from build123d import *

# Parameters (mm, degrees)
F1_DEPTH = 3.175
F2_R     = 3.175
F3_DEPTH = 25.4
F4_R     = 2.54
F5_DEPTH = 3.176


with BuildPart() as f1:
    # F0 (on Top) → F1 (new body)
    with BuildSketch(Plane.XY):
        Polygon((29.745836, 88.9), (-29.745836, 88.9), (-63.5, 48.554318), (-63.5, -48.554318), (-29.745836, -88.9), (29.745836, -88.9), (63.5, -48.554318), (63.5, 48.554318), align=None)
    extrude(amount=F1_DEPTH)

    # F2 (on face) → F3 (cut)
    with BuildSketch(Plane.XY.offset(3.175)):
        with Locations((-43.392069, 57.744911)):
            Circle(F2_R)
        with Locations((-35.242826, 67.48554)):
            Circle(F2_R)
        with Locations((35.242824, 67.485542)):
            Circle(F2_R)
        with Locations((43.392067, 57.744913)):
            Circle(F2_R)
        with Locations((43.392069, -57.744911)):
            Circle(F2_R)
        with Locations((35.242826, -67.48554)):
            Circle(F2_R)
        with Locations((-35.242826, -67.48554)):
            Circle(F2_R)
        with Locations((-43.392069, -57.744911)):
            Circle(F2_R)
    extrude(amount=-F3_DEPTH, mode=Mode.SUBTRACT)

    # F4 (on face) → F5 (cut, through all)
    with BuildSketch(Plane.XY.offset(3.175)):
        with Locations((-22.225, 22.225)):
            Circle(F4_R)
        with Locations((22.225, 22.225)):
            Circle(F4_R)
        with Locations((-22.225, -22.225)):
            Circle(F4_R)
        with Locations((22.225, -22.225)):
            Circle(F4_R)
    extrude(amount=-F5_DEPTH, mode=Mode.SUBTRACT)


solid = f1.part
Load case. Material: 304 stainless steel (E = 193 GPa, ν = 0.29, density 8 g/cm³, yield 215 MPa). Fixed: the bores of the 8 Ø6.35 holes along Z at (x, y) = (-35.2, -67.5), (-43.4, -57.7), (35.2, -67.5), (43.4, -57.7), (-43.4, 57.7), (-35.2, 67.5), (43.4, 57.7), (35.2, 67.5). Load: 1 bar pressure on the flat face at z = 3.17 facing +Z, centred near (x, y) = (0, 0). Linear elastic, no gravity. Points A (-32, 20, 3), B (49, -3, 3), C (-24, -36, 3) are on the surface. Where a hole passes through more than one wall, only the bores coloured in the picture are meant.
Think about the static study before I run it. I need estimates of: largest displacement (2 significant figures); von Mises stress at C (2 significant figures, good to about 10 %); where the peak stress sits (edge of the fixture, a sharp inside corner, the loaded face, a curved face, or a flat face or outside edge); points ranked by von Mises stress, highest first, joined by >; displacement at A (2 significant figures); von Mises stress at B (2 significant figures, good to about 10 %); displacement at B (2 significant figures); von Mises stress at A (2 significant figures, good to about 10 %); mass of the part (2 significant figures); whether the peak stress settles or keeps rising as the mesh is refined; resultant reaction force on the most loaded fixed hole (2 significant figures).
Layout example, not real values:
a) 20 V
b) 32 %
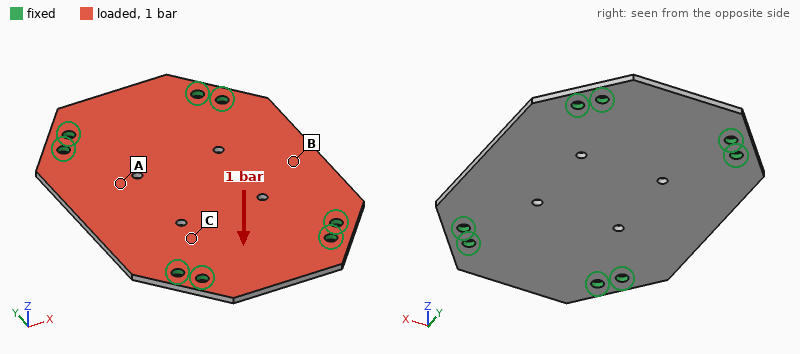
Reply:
a) 0.13 mm
b) 10 MPa
c) edge of the fixture
d) B > A > C
e) 0.093 mm
f) 36 MPa
g) 0.11 mm
h) 26 MPa
i) 500 g
j) keeps rising
k) 370 N
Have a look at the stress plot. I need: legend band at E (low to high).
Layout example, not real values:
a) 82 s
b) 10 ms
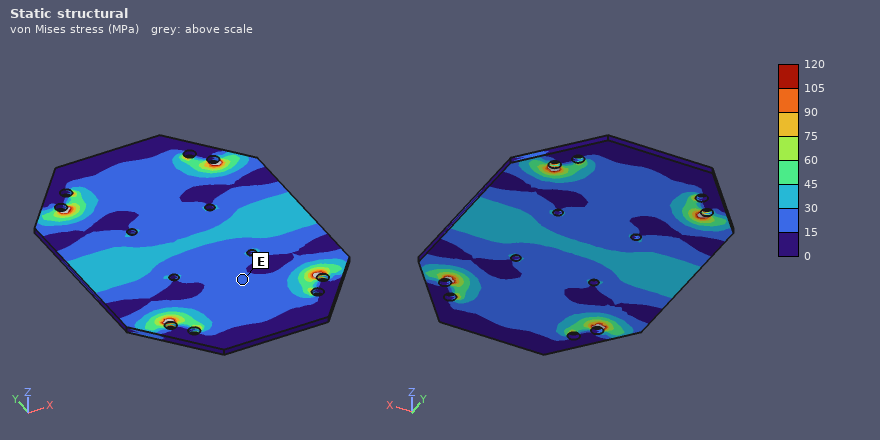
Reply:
a) 15 to 30 MPa
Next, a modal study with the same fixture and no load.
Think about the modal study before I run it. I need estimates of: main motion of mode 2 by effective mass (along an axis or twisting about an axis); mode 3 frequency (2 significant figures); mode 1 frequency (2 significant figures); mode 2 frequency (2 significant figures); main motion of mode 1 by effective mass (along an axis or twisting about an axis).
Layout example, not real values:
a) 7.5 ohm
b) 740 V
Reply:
a) twisting about Y
b) 1800 Hz
c) 1000 Hz
d) 1300 Hz
e) along Z
